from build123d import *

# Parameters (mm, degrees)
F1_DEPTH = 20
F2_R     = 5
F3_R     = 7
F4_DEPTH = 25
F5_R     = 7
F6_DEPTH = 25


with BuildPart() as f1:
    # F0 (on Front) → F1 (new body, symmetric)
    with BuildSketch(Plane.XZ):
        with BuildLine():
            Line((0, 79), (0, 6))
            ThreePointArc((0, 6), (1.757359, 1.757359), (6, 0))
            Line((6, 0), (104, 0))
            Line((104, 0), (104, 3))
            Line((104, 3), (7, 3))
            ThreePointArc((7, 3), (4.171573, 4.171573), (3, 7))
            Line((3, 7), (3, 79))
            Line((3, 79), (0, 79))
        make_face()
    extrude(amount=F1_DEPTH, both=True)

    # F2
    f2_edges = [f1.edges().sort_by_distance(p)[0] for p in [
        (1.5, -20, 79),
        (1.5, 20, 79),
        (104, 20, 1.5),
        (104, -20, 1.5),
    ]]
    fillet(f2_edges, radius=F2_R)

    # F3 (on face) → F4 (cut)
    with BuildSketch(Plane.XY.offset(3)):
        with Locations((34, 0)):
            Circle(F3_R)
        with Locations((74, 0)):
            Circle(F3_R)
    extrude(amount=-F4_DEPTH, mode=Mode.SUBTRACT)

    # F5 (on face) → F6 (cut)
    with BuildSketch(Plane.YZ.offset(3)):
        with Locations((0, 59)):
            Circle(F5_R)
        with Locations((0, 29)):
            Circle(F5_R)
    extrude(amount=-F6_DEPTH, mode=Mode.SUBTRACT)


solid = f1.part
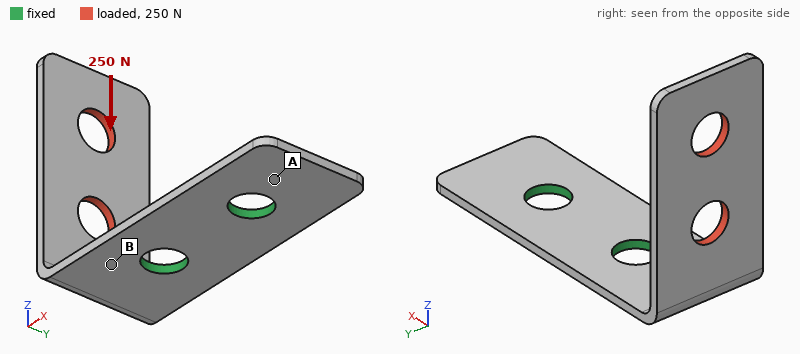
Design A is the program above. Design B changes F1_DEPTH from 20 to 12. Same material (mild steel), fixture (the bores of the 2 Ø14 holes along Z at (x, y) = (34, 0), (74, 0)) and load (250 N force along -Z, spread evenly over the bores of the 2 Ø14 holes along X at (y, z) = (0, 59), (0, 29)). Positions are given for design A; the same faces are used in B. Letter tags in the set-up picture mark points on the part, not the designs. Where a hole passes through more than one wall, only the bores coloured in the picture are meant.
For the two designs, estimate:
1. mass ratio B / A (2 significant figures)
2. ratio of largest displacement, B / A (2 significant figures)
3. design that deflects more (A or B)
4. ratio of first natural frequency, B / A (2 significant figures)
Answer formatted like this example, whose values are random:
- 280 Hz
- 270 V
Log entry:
- 0.56
- 1.5
- B
- 1.0
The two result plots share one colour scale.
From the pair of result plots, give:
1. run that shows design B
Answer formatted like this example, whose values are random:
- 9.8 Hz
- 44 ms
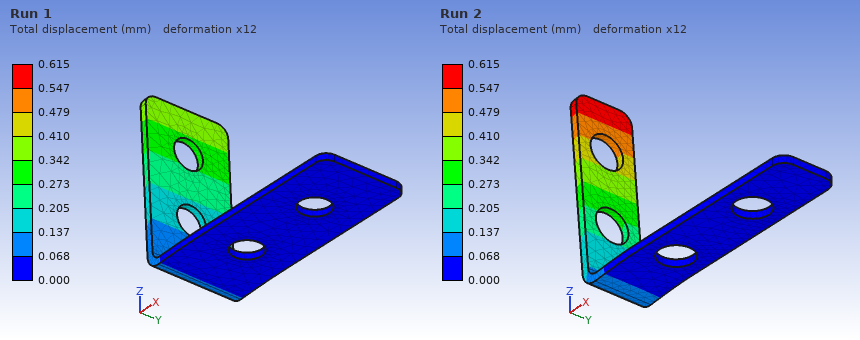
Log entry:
- Run 2
